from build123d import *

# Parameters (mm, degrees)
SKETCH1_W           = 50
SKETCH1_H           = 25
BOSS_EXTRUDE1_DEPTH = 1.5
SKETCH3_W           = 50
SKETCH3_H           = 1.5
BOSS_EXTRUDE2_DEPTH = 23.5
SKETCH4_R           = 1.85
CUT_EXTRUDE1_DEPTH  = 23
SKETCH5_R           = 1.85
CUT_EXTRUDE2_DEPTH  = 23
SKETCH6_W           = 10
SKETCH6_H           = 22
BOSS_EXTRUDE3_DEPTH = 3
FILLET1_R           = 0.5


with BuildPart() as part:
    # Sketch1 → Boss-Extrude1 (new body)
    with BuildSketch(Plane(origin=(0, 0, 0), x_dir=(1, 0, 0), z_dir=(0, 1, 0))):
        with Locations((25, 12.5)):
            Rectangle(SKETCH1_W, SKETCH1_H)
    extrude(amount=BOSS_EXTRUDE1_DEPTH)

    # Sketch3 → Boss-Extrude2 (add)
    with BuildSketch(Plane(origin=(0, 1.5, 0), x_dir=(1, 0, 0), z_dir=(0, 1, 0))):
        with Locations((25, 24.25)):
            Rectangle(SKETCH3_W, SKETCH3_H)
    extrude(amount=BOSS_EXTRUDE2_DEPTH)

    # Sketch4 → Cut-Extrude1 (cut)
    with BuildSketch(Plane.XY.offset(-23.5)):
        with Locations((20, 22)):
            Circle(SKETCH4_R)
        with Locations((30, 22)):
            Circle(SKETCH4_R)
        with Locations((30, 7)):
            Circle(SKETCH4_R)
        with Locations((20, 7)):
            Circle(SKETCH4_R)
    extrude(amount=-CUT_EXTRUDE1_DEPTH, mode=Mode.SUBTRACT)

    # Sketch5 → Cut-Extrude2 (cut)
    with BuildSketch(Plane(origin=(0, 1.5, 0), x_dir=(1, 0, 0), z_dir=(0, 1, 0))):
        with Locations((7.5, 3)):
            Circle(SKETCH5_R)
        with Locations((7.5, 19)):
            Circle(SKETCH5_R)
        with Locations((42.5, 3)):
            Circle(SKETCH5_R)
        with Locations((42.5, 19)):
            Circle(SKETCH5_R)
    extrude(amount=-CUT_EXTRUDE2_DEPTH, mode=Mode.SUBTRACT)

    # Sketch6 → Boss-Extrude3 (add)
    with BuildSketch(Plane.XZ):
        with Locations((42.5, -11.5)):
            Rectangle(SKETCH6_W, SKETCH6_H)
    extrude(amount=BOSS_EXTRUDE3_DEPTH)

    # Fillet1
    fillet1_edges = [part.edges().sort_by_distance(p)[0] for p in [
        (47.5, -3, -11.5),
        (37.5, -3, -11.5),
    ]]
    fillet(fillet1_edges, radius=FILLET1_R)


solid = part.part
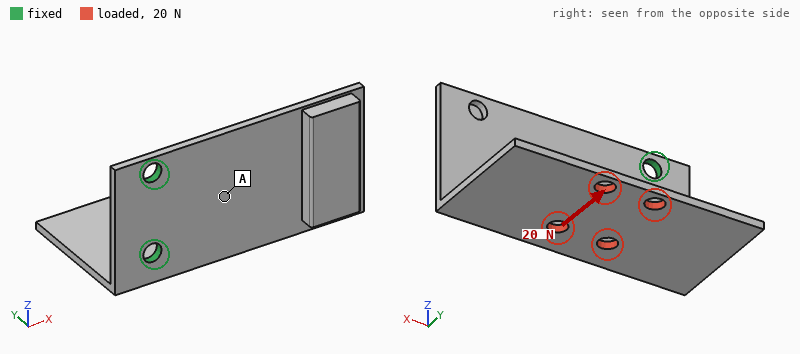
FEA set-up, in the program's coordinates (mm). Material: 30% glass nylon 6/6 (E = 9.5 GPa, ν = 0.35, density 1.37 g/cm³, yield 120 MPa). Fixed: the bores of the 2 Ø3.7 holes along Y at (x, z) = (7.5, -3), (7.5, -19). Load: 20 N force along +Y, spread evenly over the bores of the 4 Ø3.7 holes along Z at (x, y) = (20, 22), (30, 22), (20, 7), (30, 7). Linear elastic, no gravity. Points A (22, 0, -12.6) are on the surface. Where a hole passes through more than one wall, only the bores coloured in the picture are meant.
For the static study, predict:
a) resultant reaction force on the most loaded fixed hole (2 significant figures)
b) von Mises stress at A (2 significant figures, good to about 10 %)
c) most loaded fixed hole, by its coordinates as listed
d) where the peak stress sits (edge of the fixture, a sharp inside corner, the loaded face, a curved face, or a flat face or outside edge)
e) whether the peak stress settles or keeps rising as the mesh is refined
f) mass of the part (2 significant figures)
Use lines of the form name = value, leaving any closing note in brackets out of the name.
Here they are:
resultant reaction force on the most loaded fixed hole = 22 N
von Mises stress at A = 4.5 MPa
most loaded fixed hole, by its coordinates as listed = (7.5, -19)
where the peak stress sits = edge of the fixture
whether the peak stress settles or keeps rising as the mesh is refined = keeps rising
mass of the part = 5.7 g
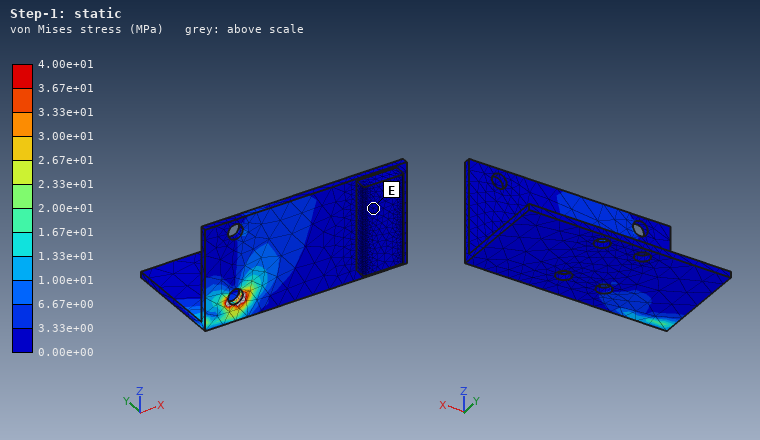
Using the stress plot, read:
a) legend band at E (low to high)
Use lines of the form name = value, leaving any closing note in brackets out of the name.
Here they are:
legend band at E = 0.00e+00 to 3.33e+00 MPa
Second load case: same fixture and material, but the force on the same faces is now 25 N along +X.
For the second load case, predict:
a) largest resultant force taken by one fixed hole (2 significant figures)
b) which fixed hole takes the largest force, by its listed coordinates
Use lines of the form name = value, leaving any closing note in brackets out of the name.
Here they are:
largest resultant force taken by one fixed hole = 30 N
which fixed hole takes the largest force, by its listed coordinates = (7.5, -19)
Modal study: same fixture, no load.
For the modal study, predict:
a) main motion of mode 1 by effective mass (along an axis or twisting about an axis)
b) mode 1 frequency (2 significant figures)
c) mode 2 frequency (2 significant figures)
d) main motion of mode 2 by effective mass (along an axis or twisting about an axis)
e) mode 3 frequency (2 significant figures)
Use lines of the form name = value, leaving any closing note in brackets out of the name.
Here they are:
main motion of mode 1 by effective mass = along Y
mode 1 frequency = 440 Hz
mode 2 frequency = 630 Hz
main motion of mode 2 by effective mass = along Z
mode 3 frequency = 1200 Hz
